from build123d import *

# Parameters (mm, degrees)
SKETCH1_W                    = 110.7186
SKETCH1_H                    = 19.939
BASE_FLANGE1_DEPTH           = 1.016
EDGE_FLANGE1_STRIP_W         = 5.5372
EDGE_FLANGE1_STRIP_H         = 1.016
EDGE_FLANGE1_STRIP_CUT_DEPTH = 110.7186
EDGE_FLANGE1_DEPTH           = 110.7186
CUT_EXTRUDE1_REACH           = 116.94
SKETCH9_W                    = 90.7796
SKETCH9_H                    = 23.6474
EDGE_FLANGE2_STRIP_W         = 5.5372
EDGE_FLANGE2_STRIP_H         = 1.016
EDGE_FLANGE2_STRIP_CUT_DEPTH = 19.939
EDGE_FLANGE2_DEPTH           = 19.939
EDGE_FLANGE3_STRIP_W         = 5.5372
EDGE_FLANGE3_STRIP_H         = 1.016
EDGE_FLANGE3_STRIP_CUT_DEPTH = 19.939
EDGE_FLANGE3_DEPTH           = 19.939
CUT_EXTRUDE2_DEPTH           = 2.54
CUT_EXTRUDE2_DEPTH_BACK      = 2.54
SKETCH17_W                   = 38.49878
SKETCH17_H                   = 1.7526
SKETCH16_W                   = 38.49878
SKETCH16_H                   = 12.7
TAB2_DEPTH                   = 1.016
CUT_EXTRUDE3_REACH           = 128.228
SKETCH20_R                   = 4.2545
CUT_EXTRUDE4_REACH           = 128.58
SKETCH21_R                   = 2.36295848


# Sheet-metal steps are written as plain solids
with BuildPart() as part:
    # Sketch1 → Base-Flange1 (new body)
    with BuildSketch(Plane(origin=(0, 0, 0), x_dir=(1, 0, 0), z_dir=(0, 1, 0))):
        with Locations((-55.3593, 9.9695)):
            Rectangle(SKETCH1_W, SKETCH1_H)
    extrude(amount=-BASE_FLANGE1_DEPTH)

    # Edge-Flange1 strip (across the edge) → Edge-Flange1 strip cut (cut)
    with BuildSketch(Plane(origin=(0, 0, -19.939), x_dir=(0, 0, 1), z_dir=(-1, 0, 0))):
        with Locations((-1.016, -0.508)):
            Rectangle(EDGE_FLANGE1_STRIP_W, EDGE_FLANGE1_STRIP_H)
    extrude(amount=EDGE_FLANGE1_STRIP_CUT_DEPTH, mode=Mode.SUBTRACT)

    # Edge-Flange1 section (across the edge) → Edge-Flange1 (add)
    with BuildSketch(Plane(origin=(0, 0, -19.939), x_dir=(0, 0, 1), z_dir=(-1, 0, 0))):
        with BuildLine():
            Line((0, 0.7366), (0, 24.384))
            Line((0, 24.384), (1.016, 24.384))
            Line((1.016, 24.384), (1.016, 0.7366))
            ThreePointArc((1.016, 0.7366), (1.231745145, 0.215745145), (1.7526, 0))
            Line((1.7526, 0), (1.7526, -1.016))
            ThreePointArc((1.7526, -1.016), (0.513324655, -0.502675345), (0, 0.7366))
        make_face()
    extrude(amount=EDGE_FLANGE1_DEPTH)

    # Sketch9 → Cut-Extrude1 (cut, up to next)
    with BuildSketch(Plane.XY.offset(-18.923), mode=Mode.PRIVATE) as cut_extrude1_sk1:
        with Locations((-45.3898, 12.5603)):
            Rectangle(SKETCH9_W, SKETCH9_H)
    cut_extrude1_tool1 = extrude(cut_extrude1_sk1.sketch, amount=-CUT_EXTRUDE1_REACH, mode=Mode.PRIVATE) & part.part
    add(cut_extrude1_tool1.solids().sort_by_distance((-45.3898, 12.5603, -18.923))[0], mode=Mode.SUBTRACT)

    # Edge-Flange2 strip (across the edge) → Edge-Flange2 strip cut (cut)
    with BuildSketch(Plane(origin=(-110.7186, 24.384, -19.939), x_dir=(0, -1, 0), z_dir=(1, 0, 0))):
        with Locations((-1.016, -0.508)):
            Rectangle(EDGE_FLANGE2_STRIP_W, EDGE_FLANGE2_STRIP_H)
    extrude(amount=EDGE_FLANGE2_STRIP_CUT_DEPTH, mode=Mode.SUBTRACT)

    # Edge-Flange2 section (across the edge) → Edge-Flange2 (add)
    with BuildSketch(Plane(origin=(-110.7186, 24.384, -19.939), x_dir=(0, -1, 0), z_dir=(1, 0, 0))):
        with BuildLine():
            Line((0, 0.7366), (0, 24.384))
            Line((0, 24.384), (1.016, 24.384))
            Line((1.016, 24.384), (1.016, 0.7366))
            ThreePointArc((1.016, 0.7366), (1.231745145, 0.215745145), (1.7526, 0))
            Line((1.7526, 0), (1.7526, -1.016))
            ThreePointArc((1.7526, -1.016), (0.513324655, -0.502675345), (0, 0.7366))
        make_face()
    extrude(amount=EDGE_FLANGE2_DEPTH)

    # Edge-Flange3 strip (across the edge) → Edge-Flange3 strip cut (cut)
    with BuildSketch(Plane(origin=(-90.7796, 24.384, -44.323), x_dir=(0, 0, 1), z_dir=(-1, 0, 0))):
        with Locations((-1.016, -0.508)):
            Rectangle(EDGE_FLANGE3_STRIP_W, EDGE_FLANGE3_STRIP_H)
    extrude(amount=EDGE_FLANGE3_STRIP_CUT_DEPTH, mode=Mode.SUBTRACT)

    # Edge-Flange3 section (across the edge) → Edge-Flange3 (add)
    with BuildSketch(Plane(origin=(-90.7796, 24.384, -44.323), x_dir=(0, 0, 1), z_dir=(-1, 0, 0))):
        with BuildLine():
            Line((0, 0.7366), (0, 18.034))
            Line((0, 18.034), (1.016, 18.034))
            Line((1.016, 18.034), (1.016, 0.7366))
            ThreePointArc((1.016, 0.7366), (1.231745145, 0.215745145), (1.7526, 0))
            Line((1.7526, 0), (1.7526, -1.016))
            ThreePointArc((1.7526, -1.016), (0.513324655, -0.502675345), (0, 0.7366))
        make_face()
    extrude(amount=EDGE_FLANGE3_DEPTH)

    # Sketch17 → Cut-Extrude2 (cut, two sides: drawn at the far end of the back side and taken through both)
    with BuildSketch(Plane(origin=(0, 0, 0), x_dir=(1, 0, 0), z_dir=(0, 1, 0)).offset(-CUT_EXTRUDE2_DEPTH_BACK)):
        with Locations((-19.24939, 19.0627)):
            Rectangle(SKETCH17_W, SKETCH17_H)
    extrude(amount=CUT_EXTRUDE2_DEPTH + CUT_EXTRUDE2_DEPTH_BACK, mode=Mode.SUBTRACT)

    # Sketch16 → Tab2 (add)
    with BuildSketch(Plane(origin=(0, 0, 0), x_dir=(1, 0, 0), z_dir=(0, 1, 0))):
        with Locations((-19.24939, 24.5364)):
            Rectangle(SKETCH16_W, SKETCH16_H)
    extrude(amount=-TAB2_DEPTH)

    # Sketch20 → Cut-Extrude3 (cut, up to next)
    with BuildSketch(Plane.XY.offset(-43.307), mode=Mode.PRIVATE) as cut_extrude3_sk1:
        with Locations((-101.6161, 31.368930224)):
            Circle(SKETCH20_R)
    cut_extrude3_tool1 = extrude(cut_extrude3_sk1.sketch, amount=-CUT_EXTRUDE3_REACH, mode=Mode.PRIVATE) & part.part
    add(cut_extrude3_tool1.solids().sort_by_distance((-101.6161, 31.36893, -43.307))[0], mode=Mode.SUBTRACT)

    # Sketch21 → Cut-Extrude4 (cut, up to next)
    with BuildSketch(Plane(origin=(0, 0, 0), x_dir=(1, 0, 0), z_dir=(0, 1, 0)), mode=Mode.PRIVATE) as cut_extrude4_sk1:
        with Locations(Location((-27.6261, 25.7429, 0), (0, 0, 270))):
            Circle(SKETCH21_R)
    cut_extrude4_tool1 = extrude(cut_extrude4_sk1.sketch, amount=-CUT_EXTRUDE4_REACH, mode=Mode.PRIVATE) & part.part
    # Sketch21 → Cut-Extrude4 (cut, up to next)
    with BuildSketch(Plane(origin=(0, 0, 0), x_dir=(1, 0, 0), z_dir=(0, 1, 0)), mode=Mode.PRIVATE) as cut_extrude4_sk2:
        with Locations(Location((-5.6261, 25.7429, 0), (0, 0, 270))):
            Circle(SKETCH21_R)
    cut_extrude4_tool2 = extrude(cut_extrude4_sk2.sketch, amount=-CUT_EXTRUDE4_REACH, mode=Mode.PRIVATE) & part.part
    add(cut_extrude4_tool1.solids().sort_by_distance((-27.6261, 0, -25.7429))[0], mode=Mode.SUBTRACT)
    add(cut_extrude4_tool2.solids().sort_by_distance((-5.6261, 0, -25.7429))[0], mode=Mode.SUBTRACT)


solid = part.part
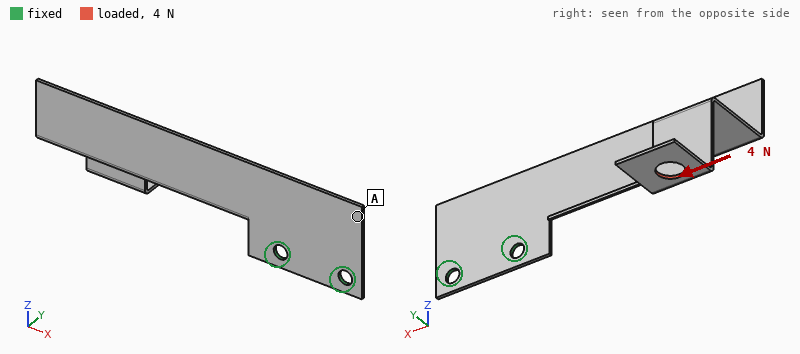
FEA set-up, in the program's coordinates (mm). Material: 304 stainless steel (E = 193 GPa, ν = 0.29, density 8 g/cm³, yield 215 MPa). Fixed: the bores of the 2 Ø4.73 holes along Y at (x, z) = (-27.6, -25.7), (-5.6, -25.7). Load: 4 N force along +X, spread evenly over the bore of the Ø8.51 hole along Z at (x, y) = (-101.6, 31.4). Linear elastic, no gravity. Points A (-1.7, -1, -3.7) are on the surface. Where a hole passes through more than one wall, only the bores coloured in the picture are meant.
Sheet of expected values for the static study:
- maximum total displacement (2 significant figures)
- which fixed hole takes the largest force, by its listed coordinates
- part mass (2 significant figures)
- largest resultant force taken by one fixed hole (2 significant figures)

1.5 mm
(-27.6, -25.7)
31 g
6.7 N
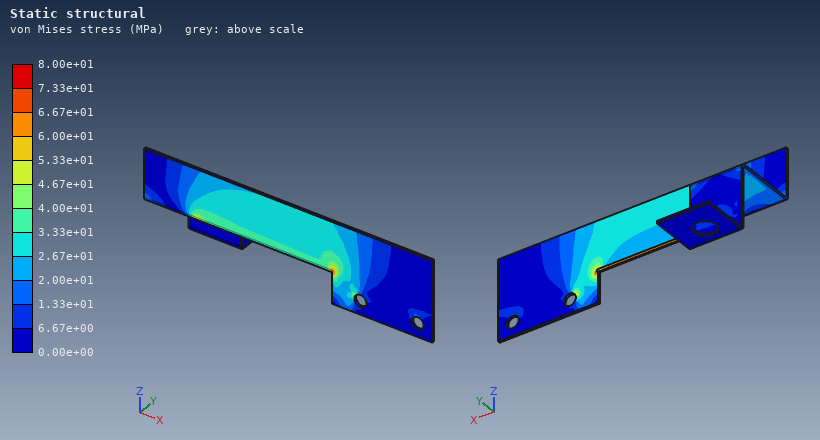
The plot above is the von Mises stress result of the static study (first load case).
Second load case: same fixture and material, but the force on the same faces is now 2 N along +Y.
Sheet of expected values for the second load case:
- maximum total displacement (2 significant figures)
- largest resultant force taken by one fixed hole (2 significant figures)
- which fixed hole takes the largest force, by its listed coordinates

1.4 mm
4.3 N
(-27.6, -25.7)
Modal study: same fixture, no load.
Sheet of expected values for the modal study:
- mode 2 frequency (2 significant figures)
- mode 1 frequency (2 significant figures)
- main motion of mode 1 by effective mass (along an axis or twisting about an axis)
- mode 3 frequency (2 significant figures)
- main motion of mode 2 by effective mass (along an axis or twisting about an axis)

130 Hz
64 Hz
along Y
300 Hz
along Z
